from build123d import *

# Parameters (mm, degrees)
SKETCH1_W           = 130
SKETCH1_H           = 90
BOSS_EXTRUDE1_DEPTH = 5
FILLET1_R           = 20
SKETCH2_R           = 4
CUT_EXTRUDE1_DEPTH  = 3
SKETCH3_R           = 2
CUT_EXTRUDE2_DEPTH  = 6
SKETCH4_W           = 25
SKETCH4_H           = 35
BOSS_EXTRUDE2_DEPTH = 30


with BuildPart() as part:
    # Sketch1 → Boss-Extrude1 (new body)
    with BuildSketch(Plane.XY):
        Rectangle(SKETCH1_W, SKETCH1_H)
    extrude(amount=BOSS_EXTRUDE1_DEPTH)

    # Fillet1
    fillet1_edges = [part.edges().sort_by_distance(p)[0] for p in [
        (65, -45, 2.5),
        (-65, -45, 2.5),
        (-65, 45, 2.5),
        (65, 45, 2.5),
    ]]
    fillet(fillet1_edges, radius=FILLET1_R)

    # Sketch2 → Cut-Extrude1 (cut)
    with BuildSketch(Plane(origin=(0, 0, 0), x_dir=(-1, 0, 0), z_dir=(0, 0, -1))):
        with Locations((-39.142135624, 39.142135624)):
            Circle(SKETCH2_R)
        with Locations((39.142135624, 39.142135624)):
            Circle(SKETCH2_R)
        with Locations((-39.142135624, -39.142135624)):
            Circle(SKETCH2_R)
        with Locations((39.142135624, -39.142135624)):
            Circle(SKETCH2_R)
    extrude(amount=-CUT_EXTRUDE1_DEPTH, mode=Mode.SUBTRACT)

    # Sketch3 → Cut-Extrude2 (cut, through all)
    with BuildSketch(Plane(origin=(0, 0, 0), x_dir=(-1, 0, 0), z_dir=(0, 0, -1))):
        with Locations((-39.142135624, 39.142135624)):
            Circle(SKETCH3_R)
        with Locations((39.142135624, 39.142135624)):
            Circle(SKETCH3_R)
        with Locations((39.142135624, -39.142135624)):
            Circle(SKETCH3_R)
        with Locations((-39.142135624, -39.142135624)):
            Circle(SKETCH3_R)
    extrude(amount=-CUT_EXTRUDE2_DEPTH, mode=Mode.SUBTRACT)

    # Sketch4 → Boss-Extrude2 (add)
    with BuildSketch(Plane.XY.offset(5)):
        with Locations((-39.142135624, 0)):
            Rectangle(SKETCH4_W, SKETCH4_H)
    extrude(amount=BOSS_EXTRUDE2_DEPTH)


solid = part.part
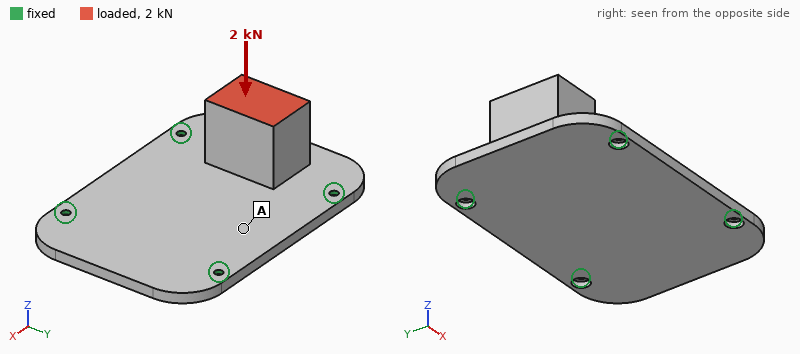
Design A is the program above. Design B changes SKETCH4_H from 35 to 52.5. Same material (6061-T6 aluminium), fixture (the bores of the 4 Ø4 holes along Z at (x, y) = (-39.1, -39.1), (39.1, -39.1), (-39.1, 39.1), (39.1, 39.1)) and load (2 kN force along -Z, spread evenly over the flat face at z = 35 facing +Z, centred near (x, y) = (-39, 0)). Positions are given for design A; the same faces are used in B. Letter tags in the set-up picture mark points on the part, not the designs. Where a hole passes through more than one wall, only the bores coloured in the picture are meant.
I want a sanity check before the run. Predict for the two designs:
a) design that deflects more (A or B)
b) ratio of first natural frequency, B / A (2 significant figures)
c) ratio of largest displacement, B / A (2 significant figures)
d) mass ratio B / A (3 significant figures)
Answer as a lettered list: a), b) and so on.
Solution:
a) A
b) 0.95
c) 0.43
d) 1.16
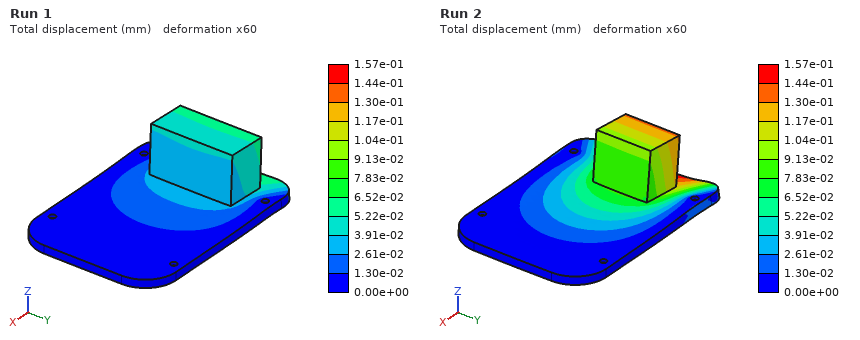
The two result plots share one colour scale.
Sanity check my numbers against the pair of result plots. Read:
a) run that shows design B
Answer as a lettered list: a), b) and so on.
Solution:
a) Run 1
